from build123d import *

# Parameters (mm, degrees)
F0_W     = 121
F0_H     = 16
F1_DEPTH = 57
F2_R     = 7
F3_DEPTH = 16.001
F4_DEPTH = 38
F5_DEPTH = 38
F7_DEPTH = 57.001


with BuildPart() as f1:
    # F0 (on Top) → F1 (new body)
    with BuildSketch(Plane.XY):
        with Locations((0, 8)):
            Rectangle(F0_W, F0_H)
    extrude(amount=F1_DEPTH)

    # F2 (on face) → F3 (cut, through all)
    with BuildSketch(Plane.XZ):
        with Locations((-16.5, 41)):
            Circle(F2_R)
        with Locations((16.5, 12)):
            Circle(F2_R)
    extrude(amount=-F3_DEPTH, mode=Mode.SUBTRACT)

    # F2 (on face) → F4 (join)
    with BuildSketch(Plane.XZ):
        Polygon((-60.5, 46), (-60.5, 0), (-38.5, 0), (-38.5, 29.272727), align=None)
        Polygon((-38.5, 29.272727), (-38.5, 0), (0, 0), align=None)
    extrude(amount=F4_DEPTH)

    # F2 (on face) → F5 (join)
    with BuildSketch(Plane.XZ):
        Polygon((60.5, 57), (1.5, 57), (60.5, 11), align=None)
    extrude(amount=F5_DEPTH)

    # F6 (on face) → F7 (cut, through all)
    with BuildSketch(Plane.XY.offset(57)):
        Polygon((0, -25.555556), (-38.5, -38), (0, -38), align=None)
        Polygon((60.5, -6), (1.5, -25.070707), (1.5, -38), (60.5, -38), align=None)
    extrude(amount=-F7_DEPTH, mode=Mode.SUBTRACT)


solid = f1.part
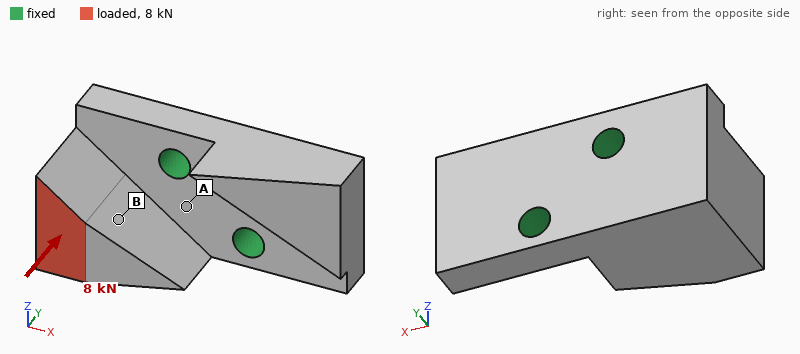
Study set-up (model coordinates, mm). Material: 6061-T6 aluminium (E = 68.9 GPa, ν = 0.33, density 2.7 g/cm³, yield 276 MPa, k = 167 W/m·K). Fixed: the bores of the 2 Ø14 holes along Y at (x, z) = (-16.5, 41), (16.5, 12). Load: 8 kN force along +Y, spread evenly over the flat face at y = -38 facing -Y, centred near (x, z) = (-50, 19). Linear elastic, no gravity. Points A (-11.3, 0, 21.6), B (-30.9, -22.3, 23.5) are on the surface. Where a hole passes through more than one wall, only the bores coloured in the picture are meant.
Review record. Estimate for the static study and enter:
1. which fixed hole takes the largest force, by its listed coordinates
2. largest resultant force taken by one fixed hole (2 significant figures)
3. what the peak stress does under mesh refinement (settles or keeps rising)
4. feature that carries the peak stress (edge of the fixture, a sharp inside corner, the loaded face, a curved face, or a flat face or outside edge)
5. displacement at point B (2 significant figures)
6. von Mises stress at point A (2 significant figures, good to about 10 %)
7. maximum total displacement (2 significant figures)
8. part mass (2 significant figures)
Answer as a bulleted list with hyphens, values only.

- (-16.5, 41)
- 8.6 kN
- keeps rising
- edge of the fixture
- 0.12 mm
- 57 MPa
- 0.27 mm
- 470 g
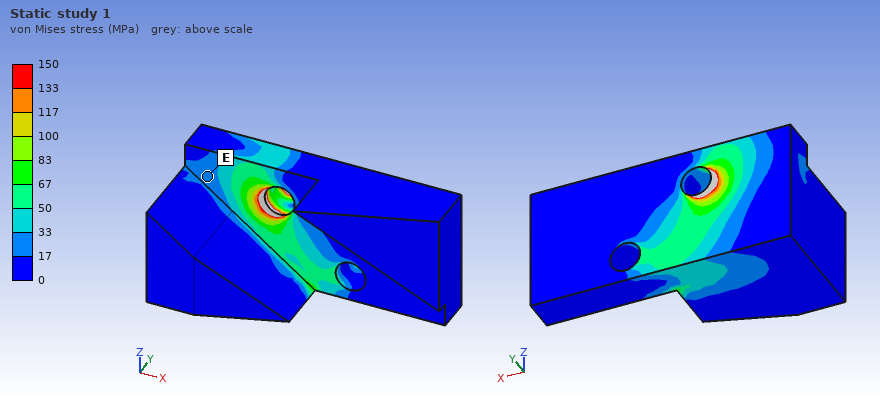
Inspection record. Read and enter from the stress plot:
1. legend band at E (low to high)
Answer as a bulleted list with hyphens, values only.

- 17 to 33 MPa
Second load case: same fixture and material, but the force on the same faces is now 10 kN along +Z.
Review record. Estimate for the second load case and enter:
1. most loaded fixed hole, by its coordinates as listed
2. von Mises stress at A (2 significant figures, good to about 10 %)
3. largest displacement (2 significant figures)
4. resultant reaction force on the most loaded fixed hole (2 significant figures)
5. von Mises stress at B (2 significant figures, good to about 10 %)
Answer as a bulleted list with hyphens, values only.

- (-16.5, 41)
- 97 MPa
- 0.49 mm
- 14 kN
- 29 MPa
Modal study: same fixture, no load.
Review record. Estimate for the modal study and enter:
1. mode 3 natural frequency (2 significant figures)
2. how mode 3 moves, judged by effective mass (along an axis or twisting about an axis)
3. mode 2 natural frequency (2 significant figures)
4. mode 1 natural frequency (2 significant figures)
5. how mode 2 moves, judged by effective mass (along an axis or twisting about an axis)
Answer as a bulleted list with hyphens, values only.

- 4600 Hz
- along Z
- 4000 Hz
- 2400 Hz
- along Y
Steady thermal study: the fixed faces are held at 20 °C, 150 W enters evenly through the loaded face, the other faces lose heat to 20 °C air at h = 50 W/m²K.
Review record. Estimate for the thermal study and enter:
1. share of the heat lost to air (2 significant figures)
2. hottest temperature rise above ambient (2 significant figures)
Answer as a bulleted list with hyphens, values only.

- 12 %
- 57 K
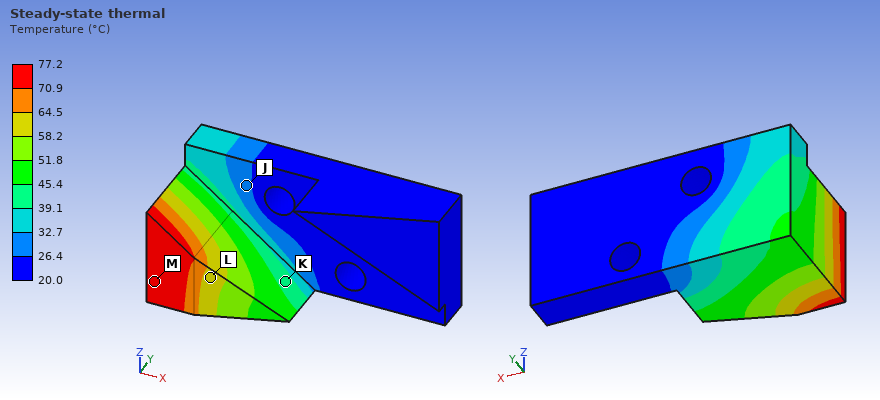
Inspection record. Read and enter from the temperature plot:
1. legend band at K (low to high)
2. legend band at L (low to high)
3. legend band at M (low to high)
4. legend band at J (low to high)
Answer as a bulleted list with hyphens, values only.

- 39.1 to 45.4 °C
- 58.2 to 64.5 °C
- 70.9 to 77.2 °C
- 26.4 to 32.7 °C
